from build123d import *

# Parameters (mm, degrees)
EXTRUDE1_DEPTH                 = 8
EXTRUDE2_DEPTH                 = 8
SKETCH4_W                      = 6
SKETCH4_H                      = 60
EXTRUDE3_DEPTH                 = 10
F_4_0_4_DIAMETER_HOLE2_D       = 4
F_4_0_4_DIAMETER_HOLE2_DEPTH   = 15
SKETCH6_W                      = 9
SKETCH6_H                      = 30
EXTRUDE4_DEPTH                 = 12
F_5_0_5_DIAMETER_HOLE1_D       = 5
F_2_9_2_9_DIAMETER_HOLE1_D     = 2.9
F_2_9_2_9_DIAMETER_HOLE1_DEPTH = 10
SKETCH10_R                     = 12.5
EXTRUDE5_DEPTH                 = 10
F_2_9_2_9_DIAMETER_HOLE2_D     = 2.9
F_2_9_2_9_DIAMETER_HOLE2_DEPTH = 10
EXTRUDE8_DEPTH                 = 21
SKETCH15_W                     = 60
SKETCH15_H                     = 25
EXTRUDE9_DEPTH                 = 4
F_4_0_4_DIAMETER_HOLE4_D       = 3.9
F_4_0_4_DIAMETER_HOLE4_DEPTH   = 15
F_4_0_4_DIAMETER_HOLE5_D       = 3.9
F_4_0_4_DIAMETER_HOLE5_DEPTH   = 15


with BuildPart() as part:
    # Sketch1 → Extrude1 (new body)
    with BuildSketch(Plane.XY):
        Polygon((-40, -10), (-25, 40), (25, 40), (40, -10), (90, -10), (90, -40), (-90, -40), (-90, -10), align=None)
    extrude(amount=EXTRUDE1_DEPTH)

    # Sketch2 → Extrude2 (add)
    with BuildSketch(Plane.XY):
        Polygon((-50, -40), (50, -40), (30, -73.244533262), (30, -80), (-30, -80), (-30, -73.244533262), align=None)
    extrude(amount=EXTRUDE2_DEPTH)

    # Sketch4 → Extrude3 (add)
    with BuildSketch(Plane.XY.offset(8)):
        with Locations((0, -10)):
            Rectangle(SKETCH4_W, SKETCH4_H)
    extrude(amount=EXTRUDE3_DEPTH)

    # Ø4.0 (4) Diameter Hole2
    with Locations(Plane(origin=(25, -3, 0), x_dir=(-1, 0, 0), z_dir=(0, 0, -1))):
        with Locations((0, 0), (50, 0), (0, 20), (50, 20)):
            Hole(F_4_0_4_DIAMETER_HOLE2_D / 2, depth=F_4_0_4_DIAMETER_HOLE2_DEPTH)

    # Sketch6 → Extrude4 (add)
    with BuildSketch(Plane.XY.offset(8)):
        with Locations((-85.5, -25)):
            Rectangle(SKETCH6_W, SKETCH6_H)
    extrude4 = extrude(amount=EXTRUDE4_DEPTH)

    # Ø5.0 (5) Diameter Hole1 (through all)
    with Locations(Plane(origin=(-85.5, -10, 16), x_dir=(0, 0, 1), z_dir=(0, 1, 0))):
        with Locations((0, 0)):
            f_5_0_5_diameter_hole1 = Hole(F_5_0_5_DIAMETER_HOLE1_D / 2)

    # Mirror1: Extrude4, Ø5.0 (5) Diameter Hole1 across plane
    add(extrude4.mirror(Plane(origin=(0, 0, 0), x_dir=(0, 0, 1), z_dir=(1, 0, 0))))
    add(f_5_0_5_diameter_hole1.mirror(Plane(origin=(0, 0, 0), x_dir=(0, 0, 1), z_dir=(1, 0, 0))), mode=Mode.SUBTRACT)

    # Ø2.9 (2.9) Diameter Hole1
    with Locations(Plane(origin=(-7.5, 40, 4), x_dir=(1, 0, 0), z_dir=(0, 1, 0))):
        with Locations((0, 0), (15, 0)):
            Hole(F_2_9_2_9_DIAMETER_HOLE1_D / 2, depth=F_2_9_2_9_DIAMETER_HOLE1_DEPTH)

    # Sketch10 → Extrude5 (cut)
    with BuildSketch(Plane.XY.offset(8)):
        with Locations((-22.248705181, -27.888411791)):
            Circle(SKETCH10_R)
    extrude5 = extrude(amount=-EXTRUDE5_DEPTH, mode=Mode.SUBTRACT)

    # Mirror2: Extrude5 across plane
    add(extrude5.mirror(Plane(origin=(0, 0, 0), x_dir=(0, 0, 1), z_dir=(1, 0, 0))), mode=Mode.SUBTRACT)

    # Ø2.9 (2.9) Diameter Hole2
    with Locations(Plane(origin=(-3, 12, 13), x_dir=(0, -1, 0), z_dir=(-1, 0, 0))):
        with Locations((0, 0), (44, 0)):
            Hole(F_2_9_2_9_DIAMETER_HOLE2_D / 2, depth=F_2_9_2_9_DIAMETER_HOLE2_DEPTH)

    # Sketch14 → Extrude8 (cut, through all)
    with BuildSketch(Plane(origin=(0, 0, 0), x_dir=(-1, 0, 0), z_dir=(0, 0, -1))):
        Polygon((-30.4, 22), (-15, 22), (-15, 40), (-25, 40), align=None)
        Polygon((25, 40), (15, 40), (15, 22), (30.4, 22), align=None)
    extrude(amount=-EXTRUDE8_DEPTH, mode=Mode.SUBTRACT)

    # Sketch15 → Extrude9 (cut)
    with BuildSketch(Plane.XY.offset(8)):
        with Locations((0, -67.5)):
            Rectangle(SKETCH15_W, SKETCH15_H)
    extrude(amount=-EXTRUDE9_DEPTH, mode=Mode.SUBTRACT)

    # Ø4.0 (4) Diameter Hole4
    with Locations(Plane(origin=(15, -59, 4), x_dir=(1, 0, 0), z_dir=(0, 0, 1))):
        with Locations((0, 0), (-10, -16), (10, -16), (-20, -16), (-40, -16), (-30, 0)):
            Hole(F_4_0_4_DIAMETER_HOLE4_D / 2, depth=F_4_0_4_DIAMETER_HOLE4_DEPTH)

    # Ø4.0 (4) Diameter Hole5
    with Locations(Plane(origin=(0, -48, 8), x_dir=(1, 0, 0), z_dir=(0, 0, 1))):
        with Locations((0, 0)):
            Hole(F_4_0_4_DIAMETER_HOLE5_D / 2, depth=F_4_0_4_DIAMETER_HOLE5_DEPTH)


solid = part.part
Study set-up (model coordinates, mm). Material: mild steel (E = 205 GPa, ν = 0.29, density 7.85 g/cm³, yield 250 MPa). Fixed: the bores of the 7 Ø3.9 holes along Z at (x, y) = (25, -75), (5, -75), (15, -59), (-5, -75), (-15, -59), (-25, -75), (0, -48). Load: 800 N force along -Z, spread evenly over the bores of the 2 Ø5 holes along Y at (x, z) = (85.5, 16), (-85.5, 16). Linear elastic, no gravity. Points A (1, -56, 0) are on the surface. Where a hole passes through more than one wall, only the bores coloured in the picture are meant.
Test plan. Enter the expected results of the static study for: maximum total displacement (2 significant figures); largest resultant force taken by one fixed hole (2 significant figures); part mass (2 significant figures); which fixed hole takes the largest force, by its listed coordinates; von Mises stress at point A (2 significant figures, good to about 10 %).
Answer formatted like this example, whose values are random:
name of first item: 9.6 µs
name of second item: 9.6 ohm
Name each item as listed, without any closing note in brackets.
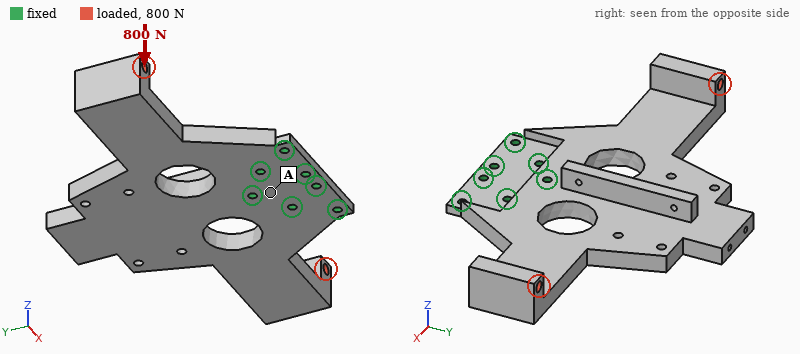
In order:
maximum total displacement: 0.25 mm
largest resultant force taken by one fixed hole: 1.0 kN
part mass: 660 g
which fixed hole takes the largest force, by its listed coordinates: (0, -48)
von Mises stress at point A: 13 MPa
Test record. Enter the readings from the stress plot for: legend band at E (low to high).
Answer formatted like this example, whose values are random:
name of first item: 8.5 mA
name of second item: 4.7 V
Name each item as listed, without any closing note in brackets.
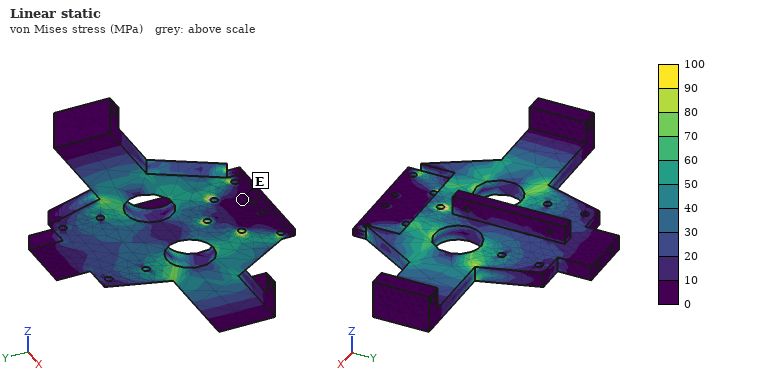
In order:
legend band at E: 0 to 10 MPa
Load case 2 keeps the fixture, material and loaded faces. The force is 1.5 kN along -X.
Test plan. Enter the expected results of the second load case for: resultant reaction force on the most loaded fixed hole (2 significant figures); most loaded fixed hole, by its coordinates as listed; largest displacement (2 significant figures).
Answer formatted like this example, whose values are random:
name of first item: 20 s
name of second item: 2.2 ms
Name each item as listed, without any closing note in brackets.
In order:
resultant reaction force on the most loaded fixed hole: 1.7 kN
most loaded fixed hole, by its coordinates as listed: (0, -48)
largest displacement: 0.14 mm
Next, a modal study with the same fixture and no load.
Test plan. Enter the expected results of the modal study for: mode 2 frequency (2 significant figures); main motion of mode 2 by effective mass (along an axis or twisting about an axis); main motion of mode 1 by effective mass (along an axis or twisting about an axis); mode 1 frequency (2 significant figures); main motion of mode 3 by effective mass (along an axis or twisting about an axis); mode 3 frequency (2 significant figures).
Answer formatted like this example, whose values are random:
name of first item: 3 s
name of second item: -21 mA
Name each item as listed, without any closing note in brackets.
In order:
mode 2 frequency: 740 Hz
main motion of mode 2 by effective mass: along Z
main motion of mode 1 by effective mass: twisting about Y
mode 1 frequency: 650 Hz
main motion of mode 3 by effective mass: twisting about X
mode 3 frequency: 1100 Hz
